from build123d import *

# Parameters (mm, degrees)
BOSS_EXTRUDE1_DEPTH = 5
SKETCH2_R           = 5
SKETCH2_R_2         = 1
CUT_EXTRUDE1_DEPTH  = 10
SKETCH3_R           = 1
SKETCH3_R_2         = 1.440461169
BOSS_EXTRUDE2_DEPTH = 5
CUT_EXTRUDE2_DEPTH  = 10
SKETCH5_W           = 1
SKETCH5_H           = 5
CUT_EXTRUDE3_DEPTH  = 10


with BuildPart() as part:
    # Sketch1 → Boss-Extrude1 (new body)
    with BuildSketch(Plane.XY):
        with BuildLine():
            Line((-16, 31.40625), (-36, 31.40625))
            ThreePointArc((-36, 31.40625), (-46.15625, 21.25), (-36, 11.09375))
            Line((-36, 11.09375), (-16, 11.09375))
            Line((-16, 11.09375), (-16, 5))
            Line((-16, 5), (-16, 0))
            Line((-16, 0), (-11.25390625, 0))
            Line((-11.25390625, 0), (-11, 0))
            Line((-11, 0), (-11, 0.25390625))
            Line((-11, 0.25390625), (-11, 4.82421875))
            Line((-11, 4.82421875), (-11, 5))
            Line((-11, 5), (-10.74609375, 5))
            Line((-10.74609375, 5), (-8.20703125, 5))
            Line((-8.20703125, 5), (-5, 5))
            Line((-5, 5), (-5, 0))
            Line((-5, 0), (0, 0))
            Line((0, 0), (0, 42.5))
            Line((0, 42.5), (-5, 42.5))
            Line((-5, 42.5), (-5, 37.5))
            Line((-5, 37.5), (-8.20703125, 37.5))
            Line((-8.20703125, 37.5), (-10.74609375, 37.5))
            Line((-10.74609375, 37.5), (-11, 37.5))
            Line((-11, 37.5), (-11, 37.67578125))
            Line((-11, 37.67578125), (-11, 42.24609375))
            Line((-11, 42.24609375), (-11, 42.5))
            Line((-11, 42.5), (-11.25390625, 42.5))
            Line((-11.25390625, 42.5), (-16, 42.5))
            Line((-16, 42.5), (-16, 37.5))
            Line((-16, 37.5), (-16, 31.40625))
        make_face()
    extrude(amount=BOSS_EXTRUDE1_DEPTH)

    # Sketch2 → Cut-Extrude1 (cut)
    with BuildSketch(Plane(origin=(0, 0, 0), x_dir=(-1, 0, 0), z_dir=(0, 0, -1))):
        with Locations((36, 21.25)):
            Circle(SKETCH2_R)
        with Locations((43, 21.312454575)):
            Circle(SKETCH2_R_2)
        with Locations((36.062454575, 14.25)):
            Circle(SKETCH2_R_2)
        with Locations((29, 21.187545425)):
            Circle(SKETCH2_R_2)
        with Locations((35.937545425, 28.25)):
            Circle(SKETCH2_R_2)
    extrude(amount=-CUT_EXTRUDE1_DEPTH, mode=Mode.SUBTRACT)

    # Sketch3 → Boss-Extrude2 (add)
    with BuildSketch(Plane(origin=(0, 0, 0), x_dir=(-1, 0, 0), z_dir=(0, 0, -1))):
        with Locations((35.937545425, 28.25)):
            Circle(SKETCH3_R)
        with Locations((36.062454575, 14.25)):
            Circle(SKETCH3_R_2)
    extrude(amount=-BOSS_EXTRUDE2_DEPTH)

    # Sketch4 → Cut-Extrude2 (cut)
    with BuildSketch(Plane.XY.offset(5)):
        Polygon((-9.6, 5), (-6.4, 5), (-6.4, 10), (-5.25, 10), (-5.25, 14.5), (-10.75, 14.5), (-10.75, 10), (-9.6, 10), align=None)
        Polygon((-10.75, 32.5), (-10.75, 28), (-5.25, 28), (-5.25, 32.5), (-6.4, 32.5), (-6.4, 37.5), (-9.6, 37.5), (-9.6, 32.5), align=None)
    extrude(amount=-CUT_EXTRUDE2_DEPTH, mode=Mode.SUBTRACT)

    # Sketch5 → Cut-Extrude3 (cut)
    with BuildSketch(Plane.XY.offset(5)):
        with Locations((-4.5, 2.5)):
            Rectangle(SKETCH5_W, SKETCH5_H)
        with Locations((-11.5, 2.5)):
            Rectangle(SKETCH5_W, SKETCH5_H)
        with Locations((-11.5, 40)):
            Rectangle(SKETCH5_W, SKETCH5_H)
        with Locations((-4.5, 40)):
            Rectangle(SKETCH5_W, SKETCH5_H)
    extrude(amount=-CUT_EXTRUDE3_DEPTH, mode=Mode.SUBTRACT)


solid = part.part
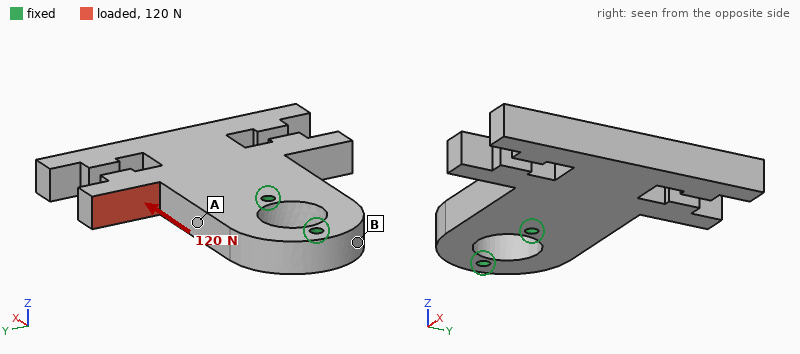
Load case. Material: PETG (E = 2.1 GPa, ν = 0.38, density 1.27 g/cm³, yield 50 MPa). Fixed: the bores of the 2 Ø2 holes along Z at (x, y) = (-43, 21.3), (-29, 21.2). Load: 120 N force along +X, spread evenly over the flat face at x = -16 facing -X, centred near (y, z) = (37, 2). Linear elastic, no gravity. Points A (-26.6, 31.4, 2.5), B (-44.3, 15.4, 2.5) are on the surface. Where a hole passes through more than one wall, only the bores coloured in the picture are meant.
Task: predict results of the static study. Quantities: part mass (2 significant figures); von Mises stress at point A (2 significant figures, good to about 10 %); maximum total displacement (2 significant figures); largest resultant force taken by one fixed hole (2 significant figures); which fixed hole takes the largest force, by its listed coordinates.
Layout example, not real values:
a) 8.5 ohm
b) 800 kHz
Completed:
a) 6.4 g
b) 7.5 MPa
c) 0.66 mm
d) 140 N
e) (-29, 21.2)
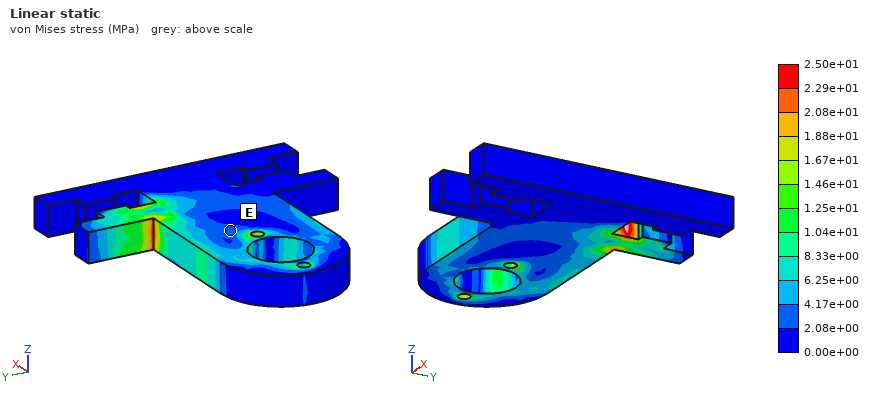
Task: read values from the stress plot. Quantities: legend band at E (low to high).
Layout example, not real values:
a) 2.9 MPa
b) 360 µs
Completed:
a) 2.08e+00 to 4.17e+00 MPa
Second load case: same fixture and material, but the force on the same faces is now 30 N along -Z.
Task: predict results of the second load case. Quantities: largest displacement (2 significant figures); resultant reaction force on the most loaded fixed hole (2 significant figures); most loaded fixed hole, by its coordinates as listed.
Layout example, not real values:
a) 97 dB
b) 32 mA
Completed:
a) 0.58 mm
b) 40 N
c) (-29, 21.2)
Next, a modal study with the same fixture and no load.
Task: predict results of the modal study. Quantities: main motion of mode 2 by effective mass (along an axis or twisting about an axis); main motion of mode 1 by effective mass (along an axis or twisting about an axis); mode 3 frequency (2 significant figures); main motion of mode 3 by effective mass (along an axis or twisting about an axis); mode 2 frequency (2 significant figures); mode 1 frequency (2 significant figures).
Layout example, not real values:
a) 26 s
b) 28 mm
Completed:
a) twisting about X
b) along Z
c) 1500 Hz
d) along Y
e) 1100 Hz
f) 830 Hz
